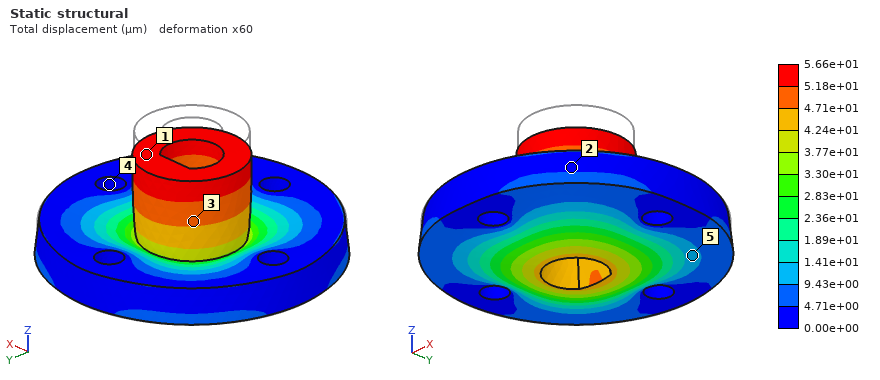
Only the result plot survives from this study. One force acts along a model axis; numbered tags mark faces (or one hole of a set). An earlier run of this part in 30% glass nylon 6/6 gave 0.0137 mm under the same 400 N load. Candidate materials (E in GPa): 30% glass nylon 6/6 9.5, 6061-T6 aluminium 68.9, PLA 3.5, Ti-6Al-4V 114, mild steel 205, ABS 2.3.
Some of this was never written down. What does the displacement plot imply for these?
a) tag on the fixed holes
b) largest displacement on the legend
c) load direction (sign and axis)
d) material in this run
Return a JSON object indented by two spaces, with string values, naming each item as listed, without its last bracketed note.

{
  "tag on the fixed holes": "4",
  "largest displacement on the legend": "5.66e+01 µm",
  "load direction": "-Z",
  "material in this run": "ABS"
}
